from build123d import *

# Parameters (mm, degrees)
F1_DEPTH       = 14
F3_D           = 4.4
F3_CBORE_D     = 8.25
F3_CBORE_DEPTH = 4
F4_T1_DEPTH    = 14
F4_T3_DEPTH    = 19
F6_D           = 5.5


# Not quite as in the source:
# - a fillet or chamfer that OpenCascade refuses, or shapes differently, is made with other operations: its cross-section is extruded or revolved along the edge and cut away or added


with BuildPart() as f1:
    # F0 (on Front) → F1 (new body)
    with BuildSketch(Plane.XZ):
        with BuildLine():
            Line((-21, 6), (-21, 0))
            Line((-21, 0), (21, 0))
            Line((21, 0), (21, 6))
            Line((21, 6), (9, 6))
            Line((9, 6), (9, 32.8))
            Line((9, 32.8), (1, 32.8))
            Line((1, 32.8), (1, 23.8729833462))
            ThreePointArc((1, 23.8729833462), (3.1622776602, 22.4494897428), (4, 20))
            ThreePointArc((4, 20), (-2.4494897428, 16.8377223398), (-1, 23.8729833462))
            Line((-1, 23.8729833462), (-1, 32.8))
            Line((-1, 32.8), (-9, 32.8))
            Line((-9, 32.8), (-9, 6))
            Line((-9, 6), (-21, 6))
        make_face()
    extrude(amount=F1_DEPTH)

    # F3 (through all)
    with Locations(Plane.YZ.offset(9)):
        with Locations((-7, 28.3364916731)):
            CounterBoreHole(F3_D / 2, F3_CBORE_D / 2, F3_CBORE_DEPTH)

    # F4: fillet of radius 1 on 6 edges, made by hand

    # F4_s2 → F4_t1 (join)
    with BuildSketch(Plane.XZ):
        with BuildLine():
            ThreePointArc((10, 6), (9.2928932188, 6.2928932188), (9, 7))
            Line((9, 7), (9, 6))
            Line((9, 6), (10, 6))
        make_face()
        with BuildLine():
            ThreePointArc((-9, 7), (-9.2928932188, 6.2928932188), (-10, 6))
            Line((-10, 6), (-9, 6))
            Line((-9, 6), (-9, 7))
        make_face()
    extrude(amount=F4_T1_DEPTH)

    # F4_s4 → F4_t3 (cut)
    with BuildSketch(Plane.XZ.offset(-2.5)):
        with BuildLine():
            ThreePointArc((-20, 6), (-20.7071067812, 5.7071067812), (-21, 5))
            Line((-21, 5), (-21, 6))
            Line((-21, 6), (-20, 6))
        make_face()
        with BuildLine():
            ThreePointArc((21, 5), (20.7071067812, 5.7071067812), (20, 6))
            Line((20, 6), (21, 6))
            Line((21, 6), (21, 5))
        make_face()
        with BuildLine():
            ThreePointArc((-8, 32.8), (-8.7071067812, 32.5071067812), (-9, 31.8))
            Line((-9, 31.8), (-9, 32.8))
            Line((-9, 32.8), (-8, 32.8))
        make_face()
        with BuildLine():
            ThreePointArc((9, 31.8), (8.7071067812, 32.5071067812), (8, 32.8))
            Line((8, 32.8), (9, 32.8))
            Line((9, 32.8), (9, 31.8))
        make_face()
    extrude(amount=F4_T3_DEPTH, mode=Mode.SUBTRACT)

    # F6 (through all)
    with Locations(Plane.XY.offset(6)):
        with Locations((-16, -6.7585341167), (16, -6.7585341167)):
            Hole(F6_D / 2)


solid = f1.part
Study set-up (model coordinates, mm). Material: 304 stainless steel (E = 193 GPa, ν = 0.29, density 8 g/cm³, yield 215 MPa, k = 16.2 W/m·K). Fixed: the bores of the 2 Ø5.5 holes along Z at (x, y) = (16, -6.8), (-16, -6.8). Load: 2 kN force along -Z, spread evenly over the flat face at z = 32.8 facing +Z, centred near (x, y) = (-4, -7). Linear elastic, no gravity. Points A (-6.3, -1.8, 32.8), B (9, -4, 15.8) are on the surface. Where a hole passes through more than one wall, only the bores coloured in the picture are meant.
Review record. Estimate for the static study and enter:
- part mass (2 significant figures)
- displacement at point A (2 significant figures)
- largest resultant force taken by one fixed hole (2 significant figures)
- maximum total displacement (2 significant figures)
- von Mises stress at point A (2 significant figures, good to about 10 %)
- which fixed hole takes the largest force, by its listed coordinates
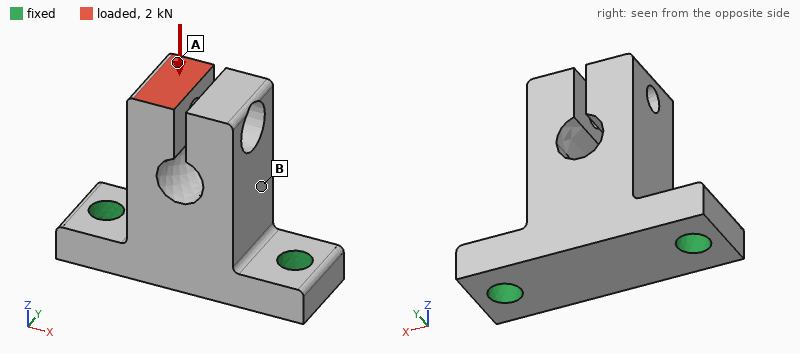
69 g
11 µm
1.4 kN
15 µm
19 MPa
(-16, -6.8)
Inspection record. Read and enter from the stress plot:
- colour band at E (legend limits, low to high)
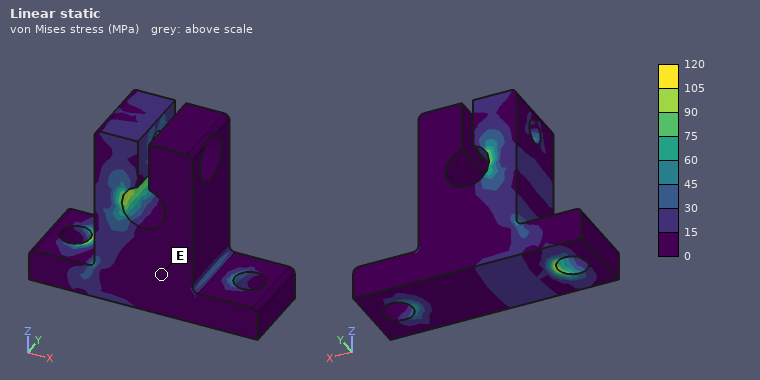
0 to 15 MPa
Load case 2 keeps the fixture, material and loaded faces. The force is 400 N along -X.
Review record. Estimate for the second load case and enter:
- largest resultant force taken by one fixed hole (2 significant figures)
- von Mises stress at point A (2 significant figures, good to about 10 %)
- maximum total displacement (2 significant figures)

570 N
8.3 MPa
30 µm
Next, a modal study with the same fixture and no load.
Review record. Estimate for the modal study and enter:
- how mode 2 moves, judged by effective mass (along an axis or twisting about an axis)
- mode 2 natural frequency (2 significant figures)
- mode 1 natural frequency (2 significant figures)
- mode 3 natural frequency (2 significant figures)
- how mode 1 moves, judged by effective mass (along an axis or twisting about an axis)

along X
8600 Hz
5300 Hz
11 kHz
along Y
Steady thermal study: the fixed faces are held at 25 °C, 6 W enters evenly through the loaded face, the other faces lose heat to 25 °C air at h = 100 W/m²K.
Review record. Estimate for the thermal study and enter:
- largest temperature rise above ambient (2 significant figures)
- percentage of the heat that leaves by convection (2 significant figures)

69 K
74 %
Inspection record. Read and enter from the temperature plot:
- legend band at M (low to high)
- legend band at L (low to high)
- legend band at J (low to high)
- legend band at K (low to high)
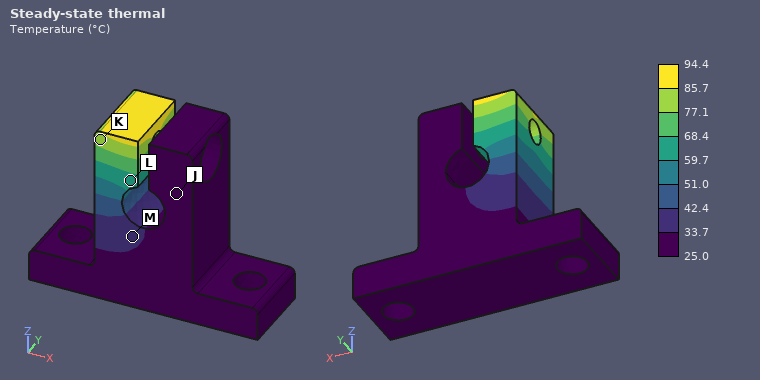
33.7 to 42.4 °C
59.7 to 68.4 °C
25.0 to 33.7 °C
77.1 to 85.7 °C
